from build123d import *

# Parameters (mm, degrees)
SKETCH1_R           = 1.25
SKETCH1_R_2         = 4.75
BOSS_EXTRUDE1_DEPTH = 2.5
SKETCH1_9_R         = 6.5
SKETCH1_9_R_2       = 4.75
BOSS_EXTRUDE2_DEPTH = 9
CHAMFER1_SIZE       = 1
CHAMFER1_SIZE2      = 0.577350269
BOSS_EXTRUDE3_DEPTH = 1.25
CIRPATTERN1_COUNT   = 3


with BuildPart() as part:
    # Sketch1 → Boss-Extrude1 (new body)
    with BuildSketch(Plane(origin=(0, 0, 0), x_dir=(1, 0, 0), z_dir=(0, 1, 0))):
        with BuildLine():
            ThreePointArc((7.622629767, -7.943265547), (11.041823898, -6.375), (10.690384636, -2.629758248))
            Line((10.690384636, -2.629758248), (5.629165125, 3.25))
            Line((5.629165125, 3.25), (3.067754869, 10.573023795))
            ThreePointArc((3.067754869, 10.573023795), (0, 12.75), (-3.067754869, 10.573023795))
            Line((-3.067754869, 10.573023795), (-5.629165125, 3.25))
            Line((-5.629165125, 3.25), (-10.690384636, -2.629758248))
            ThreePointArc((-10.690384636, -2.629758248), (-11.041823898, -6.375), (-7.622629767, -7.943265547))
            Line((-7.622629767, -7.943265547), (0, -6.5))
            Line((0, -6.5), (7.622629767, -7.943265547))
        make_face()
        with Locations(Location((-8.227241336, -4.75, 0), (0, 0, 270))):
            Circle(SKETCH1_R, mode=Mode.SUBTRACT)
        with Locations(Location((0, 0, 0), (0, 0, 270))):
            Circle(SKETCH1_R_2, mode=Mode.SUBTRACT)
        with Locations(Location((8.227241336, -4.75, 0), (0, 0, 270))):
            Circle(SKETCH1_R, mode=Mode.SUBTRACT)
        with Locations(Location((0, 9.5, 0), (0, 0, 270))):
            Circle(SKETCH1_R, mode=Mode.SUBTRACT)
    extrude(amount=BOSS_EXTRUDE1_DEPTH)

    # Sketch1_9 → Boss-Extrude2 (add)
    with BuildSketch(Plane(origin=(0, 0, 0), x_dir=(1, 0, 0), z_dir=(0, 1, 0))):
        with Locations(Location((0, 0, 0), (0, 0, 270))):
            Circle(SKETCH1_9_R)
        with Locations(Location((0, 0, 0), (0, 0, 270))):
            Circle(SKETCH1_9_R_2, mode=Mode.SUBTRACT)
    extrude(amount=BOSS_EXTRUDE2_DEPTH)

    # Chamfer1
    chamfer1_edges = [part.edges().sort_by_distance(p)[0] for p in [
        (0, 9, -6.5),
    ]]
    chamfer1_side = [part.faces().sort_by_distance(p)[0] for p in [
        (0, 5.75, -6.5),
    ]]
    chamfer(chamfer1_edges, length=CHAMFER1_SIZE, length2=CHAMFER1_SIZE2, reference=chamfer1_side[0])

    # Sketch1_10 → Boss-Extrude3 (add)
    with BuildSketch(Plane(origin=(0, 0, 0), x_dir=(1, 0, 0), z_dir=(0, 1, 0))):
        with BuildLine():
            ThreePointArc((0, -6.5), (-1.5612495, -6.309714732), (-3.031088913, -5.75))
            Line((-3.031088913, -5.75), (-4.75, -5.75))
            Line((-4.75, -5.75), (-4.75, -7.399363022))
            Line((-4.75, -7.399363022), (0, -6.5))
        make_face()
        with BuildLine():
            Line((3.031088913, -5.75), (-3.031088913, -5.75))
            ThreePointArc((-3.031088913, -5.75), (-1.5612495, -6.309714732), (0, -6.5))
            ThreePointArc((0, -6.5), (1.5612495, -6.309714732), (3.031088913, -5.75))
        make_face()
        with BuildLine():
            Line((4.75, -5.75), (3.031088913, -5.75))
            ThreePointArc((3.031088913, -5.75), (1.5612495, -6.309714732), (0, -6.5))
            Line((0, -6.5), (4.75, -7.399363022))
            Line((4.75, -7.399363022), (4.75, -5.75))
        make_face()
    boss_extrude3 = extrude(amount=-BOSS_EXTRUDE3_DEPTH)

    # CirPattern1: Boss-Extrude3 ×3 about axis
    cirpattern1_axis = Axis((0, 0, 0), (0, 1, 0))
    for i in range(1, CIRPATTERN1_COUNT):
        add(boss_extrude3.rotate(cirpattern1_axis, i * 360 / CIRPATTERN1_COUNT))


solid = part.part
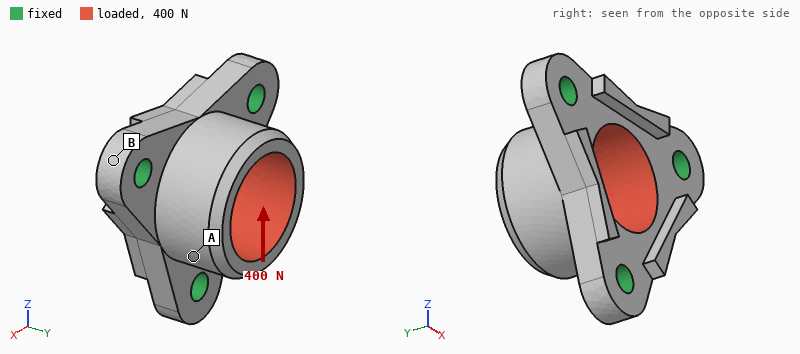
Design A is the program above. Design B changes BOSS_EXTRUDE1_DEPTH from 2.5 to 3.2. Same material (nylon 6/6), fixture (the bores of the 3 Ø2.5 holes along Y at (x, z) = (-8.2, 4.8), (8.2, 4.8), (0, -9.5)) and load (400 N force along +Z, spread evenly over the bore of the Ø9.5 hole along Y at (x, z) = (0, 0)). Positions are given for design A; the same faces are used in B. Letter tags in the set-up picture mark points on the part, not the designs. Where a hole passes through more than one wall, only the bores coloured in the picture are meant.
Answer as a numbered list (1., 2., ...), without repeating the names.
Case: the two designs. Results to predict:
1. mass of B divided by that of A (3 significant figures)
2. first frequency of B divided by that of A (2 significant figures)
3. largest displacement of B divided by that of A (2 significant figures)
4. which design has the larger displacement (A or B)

1. 1.10
2. 1.1
3. 0.76
4. A
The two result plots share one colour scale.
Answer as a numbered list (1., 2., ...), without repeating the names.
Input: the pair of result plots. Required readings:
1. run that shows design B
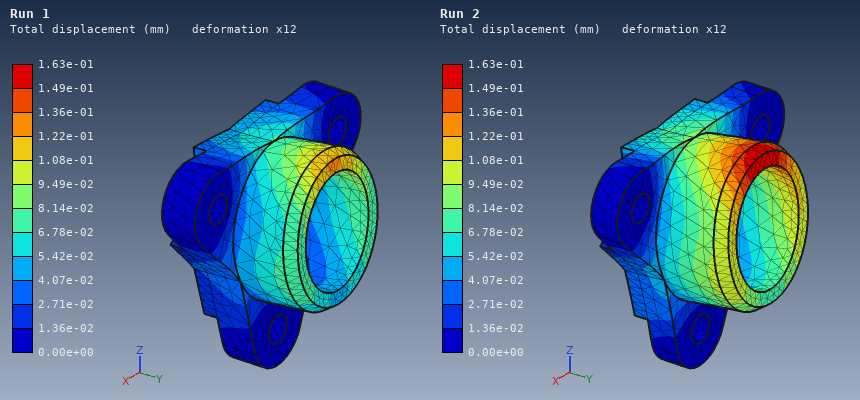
1. Run 1
